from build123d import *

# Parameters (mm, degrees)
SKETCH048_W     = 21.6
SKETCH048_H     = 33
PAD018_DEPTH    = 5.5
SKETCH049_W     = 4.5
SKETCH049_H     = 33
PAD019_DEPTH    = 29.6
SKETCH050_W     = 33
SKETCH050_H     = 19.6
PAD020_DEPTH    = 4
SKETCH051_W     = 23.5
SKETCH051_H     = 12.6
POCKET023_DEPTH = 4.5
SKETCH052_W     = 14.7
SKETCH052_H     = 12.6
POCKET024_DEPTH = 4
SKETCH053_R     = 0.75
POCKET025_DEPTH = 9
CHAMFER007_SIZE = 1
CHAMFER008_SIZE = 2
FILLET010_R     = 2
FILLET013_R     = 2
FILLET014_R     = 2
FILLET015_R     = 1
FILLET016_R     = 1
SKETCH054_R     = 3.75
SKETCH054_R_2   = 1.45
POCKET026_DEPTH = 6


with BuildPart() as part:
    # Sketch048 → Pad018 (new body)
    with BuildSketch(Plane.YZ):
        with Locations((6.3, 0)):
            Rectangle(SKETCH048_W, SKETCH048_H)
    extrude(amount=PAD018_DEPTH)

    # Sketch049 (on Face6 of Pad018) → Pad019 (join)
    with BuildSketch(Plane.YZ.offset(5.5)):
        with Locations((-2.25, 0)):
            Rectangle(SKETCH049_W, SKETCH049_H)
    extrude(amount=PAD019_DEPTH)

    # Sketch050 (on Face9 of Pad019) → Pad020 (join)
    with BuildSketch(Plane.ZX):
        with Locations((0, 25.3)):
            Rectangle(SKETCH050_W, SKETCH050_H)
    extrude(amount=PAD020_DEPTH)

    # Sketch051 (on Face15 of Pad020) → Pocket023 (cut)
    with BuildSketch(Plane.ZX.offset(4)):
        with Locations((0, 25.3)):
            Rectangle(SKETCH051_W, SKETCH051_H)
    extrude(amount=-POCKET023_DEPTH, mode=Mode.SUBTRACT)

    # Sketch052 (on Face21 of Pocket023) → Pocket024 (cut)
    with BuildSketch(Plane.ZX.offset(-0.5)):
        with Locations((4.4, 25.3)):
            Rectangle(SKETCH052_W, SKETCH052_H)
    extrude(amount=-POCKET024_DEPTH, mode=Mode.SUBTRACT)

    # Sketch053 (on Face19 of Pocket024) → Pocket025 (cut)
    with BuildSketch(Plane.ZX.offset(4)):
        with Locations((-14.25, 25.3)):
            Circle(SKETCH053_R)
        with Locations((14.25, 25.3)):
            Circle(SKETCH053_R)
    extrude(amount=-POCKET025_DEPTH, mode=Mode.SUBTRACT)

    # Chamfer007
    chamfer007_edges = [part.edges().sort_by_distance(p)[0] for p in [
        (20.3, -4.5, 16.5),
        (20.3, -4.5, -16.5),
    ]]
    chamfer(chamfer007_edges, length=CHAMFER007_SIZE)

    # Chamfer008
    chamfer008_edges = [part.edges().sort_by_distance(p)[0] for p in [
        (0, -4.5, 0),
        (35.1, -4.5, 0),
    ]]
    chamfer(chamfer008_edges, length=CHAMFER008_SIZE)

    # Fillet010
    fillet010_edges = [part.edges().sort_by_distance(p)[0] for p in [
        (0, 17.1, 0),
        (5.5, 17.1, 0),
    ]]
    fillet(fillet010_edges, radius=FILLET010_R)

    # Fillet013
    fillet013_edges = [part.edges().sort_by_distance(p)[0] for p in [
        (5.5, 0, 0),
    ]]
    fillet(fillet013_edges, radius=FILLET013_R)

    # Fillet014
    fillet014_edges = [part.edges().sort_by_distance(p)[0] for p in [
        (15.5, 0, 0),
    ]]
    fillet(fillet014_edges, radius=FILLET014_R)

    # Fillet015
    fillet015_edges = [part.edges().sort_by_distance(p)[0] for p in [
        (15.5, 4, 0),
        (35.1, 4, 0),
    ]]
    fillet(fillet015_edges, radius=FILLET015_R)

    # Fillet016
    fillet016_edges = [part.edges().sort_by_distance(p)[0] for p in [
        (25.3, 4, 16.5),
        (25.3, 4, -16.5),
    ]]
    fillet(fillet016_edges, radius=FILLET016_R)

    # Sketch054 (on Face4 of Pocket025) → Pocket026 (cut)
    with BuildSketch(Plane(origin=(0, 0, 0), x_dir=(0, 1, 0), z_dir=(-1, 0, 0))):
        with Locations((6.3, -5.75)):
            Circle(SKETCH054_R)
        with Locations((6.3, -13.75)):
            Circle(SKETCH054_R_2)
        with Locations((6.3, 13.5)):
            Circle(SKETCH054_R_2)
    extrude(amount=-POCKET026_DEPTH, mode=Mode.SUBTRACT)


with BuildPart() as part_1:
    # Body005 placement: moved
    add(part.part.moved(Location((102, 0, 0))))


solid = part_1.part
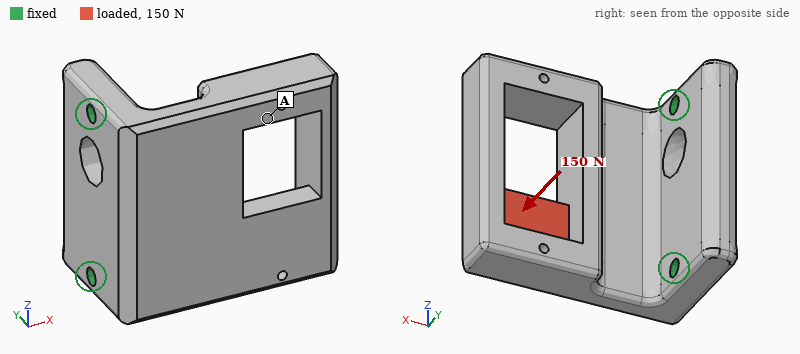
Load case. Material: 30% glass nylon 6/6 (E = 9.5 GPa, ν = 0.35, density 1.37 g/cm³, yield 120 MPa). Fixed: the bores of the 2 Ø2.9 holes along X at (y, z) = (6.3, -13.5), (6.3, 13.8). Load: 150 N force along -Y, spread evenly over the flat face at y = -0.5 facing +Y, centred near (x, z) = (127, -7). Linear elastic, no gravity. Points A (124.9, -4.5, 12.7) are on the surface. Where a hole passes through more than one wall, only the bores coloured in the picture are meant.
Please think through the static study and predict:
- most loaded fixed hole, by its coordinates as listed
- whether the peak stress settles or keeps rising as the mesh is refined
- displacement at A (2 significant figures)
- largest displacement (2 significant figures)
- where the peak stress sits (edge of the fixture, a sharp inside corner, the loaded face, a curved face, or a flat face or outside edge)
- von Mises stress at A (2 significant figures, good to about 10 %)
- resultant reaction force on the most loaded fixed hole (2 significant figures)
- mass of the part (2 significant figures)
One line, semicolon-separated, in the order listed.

(6.3, -13.5); keeps rising; 0.27 mm; 0.63 mm; edge of the fixture; 6.8 MPa; 120 N; 11 g
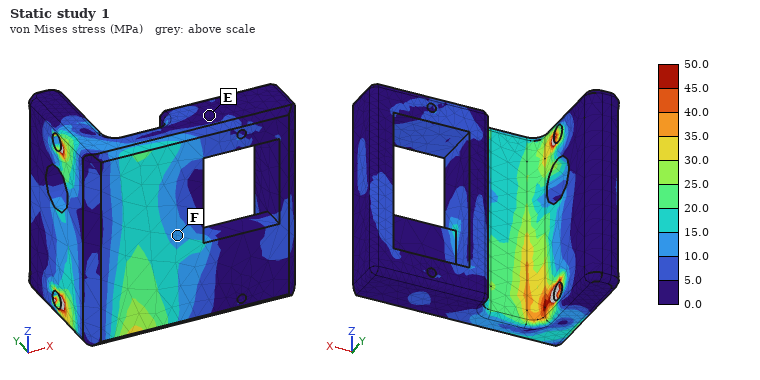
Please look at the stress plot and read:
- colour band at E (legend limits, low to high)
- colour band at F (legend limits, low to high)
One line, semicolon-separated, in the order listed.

0.0 to 5.0 MPa; 10.0 to 15.0 MPa
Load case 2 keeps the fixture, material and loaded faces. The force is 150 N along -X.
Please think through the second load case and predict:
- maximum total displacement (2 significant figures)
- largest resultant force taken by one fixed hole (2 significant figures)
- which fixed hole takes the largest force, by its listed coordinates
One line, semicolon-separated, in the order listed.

27 µm; 120 N; (6.3, -13.5)
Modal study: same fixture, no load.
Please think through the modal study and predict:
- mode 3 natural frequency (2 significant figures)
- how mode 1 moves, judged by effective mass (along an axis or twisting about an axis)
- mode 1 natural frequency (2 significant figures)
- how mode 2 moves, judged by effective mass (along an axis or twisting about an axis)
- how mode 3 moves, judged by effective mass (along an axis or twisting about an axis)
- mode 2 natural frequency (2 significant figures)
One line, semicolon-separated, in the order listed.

4300 Hz; along Y; 1400 Hz; along Z; along Z; 3100 Hz
